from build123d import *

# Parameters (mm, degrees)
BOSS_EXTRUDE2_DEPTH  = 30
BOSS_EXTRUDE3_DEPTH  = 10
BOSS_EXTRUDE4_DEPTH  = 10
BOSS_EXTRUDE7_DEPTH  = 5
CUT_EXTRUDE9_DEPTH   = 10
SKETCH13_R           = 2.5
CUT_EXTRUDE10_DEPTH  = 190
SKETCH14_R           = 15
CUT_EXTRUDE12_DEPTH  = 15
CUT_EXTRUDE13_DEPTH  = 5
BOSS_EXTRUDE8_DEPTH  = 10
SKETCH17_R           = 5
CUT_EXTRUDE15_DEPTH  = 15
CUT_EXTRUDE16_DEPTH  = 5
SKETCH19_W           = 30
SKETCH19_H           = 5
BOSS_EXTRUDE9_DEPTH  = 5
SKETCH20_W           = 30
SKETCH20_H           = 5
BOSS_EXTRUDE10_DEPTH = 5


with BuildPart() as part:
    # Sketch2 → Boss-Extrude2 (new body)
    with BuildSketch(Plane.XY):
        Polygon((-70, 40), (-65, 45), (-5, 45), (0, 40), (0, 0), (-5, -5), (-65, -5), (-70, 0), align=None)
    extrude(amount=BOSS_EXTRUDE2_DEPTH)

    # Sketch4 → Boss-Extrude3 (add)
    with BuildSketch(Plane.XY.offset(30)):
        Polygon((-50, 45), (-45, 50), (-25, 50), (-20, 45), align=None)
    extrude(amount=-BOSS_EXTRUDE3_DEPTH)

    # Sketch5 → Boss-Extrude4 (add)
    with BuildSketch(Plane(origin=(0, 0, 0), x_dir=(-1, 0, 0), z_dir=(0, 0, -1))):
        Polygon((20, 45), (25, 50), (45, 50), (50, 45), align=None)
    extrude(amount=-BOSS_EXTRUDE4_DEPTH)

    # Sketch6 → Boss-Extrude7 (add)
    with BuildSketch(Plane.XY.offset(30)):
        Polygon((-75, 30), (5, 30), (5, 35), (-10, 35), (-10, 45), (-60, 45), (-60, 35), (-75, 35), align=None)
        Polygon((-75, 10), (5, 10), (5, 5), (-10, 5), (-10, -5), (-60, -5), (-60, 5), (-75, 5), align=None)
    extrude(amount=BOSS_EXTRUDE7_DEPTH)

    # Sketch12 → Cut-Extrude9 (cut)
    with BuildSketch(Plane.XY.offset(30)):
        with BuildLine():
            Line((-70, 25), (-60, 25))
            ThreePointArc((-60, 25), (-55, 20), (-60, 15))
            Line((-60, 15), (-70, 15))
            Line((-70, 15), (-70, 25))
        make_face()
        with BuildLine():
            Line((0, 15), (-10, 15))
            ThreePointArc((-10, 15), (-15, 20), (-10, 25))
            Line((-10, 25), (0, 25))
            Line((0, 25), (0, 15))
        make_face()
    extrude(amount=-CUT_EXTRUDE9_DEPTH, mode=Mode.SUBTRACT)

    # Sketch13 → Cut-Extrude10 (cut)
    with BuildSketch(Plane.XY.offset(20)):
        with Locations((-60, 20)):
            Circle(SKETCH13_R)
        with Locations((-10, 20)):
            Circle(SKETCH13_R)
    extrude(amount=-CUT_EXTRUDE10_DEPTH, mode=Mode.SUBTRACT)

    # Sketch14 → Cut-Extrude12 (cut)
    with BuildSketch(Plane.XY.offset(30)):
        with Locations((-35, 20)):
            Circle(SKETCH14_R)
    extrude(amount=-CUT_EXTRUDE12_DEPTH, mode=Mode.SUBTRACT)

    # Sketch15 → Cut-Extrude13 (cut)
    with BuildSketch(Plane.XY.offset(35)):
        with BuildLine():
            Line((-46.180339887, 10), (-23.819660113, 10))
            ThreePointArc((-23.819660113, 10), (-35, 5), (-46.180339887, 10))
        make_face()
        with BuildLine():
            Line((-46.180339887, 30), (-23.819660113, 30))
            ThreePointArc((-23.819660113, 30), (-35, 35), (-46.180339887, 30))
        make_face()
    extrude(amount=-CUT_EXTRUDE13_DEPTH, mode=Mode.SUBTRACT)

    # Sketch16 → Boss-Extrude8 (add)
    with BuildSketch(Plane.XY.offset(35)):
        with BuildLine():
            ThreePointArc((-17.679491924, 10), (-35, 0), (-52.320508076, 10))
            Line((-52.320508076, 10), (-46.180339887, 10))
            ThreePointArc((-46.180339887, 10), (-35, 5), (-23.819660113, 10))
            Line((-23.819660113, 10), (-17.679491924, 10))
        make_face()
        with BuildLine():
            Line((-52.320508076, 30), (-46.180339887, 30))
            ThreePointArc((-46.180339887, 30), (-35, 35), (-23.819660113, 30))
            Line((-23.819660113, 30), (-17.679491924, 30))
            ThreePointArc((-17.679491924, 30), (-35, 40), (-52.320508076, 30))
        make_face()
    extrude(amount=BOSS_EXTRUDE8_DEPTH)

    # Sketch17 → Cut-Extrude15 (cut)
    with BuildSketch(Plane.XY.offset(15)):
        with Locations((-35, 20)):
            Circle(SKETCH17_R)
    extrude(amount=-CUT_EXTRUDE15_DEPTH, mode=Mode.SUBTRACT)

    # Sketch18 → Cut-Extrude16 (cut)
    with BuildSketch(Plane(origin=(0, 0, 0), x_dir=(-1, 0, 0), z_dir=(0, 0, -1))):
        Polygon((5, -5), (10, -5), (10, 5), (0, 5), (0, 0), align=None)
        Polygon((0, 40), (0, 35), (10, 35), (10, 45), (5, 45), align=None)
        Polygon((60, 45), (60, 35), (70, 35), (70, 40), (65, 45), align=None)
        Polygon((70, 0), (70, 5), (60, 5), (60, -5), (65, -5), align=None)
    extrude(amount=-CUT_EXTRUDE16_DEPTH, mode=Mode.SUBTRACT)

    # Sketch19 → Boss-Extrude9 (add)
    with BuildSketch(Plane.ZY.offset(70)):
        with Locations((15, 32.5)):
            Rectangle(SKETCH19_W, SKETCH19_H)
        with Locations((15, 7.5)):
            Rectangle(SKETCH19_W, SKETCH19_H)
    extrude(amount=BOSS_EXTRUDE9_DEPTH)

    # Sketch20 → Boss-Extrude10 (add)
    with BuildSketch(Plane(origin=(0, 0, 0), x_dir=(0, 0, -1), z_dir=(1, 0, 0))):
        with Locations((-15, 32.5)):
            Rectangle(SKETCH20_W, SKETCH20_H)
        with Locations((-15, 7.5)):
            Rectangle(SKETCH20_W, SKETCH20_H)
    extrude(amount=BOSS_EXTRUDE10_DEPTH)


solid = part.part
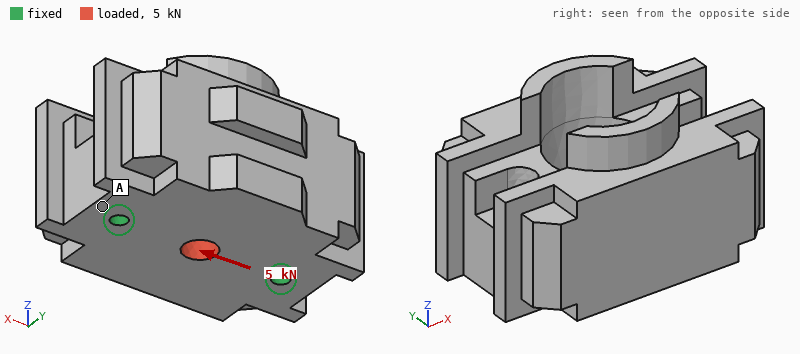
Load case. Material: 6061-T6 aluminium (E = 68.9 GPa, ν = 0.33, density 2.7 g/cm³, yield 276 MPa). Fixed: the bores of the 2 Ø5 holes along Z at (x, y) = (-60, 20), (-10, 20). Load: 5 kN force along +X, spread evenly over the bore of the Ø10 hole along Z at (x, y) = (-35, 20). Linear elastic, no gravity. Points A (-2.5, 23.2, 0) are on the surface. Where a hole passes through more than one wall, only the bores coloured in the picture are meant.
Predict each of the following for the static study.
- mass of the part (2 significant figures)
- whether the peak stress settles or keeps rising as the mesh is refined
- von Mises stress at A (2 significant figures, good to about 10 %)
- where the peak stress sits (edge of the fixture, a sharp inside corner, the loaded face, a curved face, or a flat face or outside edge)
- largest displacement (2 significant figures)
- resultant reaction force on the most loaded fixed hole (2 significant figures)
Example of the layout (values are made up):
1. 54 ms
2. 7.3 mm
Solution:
1. 280 g
2. keeps rising
3. 2.5 MPa
4. edge of the fixture
5. 2.9 µm
6. 2.5 kN
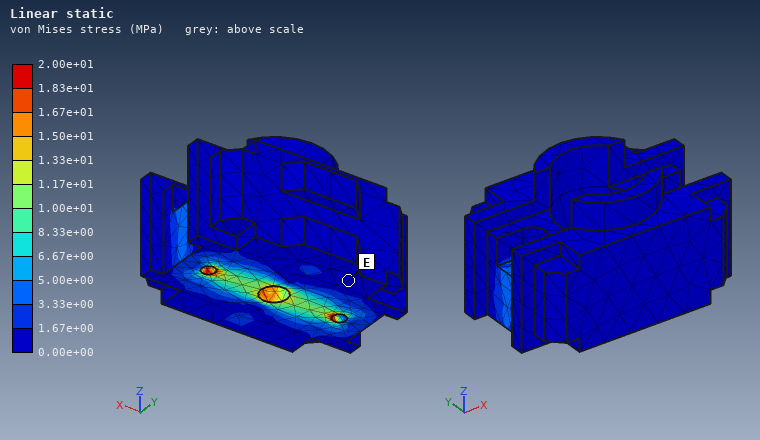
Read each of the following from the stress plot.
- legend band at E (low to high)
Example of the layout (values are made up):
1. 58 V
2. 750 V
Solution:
1. 0.00e+00 to 1.67e+00 MPa
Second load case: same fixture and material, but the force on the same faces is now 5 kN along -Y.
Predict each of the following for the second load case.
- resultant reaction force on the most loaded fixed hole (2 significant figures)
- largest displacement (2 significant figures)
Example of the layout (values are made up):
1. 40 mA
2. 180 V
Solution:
1. 2.5 kN
2. 5.0 µm
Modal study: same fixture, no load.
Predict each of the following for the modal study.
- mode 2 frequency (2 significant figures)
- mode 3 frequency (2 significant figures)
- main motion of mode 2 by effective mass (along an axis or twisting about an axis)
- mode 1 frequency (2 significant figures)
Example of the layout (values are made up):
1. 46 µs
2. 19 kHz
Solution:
1. 12 kHz
2. 14 kHz
3. along Z
4. 7700 Hz
